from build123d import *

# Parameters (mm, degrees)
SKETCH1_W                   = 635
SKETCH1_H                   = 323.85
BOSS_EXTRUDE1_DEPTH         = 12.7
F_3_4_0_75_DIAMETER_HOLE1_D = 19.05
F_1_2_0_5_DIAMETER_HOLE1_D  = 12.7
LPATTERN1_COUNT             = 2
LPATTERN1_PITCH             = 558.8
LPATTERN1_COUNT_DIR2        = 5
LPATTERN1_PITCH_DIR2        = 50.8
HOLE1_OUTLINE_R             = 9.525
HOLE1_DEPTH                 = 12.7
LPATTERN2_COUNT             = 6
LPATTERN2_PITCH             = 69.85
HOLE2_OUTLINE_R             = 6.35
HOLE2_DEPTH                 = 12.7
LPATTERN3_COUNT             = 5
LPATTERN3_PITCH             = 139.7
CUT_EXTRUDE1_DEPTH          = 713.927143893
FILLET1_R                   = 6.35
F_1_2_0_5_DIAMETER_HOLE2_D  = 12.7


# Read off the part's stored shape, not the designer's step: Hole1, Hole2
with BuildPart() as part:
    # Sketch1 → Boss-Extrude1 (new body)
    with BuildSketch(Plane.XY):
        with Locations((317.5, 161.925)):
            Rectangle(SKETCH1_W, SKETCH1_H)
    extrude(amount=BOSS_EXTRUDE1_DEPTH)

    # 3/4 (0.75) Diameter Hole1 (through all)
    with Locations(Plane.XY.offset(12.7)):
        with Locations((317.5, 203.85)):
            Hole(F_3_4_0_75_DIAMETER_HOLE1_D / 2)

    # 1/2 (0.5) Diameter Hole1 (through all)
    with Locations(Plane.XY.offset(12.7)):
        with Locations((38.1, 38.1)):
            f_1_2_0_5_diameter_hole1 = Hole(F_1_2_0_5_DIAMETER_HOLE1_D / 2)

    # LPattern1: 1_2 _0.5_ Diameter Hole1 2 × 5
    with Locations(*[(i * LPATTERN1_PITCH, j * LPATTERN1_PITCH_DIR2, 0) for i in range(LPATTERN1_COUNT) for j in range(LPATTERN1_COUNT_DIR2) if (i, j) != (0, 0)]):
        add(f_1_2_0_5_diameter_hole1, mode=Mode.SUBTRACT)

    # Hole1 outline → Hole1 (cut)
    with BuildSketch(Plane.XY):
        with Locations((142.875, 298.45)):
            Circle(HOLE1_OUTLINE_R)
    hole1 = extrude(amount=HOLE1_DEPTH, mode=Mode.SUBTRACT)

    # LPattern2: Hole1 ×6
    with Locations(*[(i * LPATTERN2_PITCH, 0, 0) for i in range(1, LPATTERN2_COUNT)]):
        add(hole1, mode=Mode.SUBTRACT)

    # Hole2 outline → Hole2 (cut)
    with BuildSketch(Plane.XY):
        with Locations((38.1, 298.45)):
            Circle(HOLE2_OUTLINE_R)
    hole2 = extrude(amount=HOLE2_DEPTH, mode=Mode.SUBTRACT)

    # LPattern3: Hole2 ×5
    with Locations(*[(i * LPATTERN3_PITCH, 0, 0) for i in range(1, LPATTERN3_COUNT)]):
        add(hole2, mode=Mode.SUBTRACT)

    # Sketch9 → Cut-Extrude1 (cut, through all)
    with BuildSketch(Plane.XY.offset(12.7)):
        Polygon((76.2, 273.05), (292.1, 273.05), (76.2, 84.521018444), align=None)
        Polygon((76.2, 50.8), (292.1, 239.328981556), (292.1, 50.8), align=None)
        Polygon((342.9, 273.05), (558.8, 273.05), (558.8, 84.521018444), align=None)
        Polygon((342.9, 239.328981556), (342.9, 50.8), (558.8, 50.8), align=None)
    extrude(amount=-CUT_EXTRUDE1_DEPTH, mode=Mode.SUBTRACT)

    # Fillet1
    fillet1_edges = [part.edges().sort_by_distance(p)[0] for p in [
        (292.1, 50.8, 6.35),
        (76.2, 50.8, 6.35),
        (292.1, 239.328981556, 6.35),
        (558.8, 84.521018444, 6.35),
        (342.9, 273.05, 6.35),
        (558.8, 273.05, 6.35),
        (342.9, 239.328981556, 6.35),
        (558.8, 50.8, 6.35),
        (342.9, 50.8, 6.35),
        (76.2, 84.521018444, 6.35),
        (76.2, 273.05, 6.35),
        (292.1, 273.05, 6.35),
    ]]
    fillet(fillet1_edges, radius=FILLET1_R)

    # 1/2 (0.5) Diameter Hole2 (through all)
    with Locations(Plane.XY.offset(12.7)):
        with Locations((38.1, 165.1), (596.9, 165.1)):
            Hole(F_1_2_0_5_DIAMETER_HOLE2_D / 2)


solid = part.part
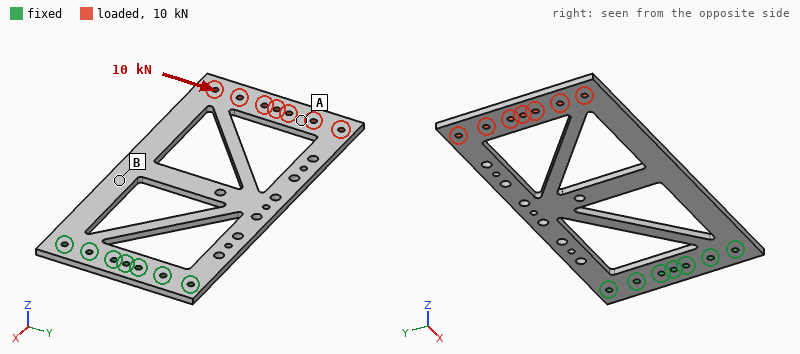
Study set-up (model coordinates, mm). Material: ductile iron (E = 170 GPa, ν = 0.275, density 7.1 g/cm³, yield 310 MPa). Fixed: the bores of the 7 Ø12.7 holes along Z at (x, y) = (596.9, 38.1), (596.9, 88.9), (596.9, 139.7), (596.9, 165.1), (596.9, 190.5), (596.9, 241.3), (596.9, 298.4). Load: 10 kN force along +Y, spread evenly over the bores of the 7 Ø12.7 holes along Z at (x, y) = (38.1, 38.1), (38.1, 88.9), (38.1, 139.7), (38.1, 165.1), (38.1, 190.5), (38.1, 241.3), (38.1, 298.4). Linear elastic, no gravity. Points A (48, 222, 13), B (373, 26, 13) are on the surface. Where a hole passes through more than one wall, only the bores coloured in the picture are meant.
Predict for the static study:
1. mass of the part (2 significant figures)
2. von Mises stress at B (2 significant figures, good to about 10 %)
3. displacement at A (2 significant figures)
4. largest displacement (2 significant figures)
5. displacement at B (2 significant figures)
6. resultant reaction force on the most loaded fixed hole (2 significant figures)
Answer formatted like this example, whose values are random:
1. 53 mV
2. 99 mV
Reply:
1. 11 kg
2. 17 MPa
3. 0.38 mm
4. 0.41 mm
5. 0.13 mm
6. 22 kN
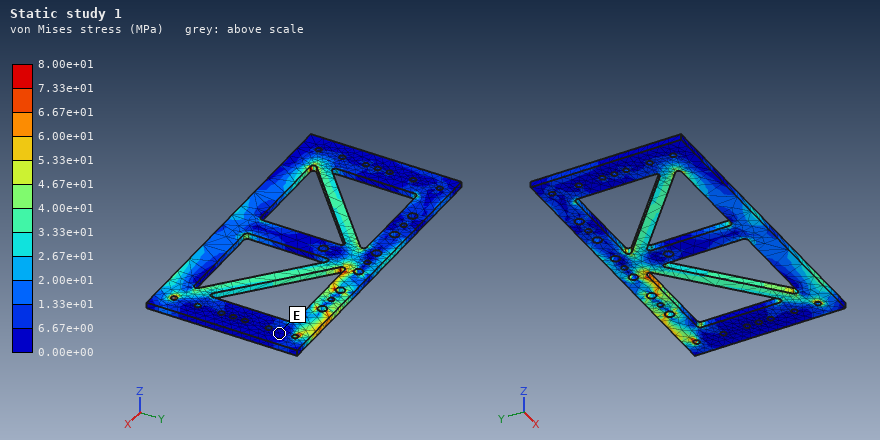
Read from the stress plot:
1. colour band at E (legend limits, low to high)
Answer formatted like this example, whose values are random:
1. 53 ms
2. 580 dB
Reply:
1. 0.00e+00 to 6.67e+00 MPa
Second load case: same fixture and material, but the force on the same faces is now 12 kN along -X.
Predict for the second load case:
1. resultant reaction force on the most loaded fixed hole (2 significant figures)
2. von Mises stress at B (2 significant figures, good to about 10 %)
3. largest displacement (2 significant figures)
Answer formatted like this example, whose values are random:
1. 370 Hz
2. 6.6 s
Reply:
1. 5.6 kN
2. 8.6 MPa
3. 62 µm
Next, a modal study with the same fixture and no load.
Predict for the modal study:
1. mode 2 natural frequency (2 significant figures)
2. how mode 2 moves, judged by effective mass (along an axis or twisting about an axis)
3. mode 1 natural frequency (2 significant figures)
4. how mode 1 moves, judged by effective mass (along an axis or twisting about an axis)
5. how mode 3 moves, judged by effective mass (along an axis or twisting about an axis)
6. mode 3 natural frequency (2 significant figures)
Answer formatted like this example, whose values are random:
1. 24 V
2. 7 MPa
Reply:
1. 84 Hz
2. twisting about X
3. 22 Hz
4. along Z
5. along Z
6. 140 Hz
